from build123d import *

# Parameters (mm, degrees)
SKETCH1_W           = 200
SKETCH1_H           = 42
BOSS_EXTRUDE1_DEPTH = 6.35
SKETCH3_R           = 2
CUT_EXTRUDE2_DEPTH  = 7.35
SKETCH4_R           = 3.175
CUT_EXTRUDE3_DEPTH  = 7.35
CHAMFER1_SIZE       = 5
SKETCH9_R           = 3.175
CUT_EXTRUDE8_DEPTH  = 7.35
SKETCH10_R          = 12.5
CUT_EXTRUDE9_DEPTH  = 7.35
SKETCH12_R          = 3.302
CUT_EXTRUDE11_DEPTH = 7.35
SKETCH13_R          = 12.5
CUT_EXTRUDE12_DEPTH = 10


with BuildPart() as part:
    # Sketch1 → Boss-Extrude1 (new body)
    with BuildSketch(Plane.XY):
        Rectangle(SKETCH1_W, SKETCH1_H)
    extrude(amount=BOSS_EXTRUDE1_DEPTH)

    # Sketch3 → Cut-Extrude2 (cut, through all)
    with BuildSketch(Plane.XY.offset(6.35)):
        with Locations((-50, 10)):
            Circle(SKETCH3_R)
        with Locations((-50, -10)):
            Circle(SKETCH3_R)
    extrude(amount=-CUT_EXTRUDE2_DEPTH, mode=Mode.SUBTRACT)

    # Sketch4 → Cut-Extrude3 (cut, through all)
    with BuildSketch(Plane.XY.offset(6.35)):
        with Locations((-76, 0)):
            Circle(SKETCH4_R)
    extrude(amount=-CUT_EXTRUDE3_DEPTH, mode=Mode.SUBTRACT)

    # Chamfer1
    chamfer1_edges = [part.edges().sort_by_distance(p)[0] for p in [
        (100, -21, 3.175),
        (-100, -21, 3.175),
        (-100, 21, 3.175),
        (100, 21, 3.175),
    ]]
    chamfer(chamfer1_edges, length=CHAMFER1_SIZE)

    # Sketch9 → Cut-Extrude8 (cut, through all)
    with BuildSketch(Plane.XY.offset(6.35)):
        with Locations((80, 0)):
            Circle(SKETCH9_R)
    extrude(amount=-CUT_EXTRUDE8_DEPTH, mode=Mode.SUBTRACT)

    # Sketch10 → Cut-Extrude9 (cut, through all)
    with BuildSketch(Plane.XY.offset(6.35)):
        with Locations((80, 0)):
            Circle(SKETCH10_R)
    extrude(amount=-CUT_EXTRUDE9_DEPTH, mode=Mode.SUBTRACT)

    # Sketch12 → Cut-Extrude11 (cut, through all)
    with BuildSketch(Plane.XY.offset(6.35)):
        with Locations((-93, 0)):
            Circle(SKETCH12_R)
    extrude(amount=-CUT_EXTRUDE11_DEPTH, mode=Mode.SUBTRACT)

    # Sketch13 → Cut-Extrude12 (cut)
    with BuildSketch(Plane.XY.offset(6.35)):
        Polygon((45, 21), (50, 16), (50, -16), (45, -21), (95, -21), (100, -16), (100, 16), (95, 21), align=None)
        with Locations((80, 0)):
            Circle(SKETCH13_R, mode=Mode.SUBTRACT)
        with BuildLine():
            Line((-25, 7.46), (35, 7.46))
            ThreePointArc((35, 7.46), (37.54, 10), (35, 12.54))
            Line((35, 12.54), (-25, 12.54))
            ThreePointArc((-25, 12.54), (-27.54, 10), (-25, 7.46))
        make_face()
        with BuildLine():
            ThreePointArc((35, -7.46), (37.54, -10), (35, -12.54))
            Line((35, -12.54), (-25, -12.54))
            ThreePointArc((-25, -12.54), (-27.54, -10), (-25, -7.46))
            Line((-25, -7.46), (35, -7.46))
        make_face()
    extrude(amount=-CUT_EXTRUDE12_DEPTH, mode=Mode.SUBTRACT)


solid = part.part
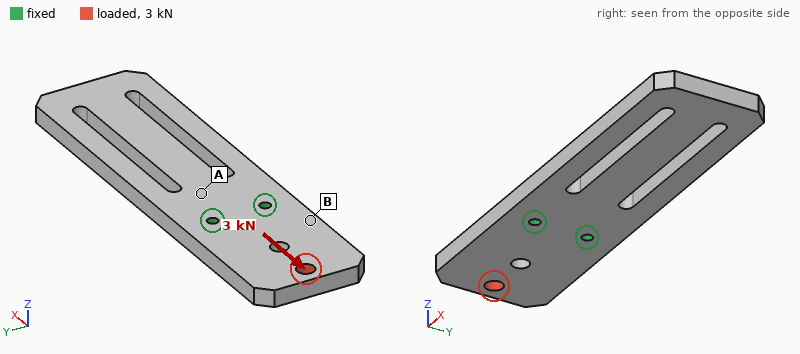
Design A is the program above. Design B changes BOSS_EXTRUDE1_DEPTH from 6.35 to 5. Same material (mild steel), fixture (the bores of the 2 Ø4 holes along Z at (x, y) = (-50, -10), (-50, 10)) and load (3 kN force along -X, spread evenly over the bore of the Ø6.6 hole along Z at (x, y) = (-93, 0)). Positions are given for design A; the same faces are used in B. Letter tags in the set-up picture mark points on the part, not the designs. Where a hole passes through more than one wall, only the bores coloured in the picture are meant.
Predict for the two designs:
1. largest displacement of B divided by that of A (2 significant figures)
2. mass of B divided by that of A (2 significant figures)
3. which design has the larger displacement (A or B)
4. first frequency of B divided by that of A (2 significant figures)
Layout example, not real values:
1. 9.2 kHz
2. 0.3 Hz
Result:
1. 1.3
2. 0.79
3. B
4. 0.79
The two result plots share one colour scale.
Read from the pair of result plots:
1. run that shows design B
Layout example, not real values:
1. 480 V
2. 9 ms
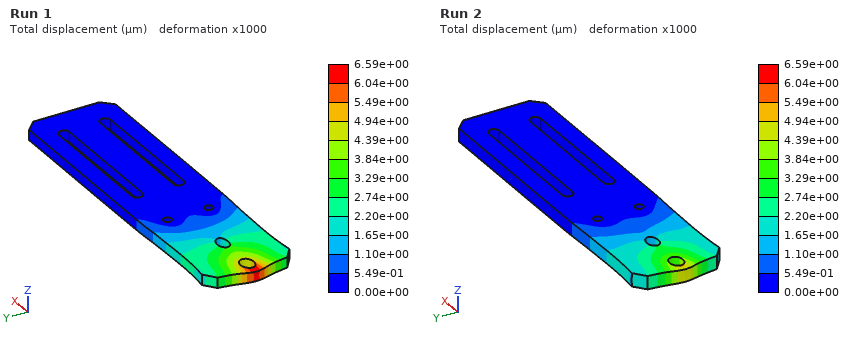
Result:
1. Run 1
